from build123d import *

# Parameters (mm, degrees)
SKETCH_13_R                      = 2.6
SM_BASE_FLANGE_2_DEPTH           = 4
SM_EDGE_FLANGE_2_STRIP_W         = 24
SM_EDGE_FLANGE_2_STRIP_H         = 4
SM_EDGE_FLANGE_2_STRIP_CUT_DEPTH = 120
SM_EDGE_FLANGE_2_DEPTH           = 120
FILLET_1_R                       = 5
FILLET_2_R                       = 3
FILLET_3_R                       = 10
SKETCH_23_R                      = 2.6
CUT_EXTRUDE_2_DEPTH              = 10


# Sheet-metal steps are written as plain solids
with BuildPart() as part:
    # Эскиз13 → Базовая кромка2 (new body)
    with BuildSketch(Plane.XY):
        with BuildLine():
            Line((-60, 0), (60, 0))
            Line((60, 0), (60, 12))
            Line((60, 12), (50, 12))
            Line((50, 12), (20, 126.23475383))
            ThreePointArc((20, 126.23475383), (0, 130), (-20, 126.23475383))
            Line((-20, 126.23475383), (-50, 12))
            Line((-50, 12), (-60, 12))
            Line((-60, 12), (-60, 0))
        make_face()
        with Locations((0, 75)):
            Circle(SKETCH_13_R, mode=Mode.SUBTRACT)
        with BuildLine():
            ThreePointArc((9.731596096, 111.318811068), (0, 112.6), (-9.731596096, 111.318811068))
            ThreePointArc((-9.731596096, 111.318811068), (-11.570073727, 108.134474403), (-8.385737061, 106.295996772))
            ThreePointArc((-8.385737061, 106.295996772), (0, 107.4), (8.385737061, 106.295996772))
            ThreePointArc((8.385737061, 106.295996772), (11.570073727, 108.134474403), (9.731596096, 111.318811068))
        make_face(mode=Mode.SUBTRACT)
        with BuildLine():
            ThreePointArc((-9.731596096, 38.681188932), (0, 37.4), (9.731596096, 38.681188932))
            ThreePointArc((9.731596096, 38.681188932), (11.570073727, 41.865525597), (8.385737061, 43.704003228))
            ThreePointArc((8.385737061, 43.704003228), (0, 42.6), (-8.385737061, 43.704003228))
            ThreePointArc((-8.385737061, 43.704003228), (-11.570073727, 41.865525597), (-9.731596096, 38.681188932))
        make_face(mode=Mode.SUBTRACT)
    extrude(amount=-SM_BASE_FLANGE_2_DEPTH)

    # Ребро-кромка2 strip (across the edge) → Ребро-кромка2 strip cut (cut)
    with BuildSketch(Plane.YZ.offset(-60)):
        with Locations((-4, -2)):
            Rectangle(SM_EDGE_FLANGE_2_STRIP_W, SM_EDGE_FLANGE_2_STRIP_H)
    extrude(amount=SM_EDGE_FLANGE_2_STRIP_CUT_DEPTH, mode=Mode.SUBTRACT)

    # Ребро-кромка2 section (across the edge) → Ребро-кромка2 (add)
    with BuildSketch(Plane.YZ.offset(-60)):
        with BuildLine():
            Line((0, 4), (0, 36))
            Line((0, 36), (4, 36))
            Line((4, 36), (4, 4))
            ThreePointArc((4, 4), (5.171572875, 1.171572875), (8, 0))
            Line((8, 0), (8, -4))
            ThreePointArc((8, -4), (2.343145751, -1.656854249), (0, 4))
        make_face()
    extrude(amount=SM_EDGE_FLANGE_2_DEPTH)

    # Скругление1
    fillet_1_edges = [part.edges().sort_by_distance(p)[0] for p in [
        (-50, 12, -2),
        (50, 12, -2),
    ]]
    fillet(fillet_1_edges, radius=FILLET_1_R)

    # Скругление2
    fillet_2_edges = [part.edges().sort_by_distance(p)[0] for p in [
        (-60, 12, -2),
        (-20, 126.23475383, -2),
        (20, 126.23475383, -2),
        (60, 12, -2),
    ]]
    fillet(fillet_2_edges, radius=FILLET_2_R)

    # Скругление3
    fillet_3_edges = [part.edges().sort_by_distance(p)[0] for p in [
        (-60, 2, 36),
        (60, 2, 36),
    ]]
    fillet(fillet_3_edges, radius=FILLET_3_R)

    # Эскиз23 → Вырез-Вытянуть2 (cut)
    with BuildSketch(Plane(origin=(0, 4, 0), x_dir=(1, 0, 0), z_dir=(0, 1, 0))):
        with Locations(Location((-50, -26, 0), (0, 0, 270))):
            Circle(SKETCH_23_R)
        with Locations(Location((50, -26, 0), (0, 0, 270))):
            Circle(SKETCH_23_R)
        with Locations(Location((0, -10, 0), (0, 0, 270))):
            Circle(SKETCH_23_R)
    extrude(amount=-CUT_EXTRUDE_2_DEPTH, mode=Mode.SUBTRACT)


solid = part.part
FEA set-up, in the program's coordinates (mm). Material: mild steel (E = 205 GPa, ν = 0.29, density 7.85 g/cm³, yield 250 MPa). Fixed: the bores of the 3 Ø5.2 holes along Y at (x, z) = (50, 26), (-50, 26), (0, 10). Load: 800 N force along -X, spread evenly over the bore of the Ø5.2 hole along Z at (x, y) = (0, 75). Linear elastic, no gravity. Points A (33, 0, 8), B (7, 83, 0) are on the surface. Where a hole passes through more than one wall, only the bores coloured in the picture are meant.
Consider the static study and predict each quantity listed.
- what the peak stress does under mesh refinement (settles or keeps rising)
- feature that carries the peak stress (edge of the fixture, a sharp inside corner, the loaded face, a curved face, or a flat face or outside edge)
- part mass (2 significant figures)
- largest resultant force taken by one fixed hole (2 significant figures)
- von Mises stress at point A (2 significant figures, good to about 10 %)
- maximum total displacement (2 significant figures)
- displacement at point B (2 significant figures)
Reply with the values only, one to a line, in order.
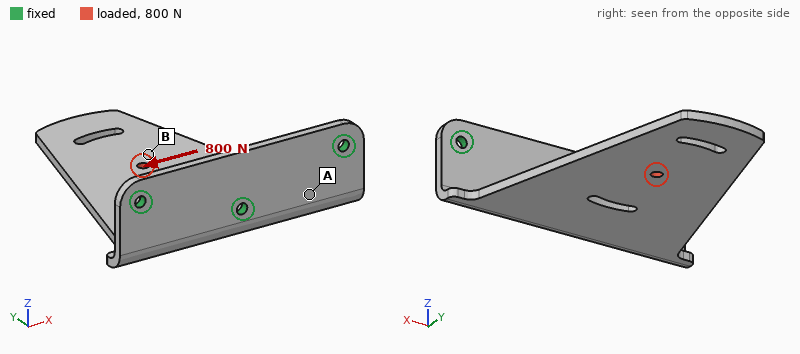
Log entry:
keeps rising
edge of the fixture
410 g
560 N
39 MPa
0.19 mm
0.12 mm
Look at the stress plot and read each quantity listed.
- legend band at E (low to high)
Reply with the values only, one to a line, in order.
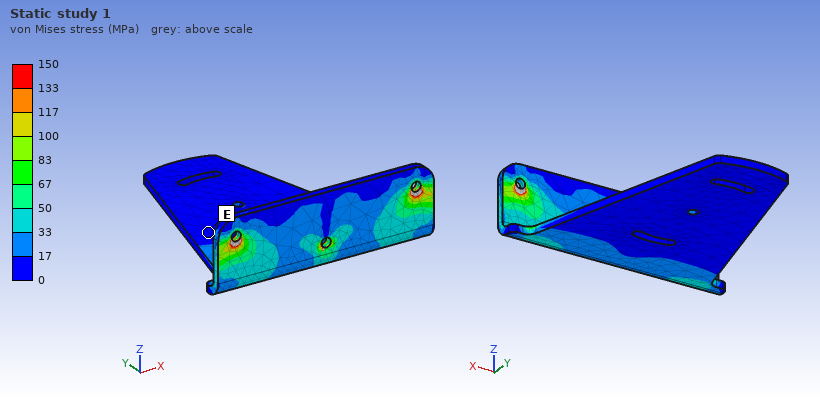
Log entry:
0 to 17 MPa
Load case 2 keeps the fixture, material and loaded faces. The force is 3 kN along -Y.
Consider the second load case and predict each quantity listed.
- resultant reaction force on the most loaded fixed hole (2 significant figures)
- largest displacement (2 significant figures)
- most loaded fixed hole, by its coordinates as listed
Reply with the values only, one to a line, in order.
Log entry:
3.0 kN
0.44 mm
(0, 10)
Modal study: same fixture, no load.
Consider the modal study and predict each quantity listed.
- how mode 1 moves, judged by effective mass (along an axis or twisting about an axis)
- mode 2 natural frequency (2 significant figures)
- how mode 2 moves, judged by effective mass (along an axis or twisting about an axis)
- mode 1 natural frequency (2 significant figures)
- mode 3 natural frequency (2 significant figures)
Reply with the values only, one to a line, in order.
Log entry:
along Z
810 Hz
along X
240 Hz
1200 Hz
